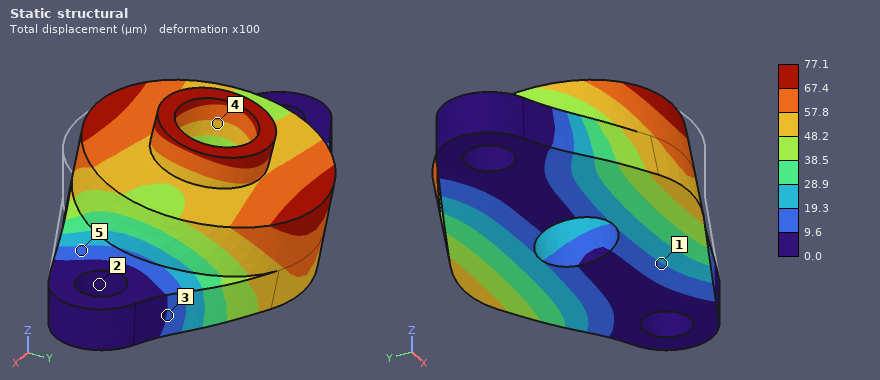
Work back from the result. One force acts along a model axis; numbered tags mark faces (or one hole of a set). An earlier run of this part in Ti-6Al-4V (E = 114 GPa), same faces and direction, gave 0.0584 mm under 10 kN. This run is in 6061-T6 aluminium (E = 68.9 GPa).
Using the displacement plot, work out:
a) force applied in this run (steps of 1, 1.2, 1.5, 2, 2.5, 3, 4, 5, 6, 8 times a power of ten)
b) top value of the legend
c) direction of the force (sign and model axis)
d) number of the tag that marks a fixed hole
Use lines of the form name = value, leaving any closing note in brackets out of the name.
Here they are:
force applied in this run = 8 kN
top value of the legend = 77.1 µm
direction of the force = +Y
number of the tag that marks a fixed hole = 2
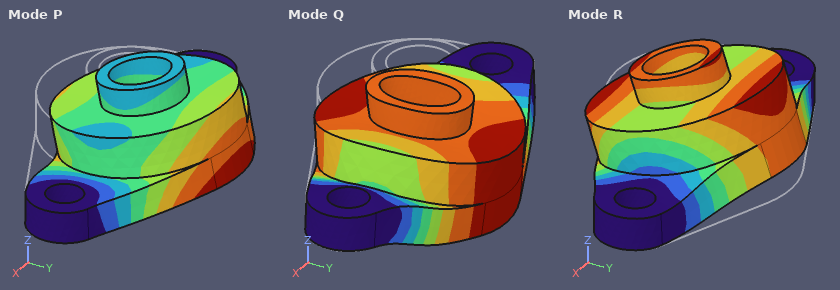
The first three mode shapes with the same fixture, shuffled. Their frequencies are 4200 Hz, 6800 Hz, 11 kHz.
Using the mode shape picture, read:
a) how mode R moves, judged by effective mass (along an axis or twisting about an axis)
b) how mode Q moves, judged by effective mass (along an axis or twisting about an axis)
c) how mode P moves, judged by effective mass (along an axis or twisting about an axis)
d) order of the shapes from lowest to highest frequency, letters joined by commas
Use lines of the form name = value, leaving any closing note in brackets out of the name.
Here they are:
how mode R moves, judged by effective mass = along Y
how mode Q moves, judged by effective mass = along Z
how mode P moves, judged by effective mass = along Y
order of the shapes from lowest to highest frequency, letters joined by commas = R, Q, P
